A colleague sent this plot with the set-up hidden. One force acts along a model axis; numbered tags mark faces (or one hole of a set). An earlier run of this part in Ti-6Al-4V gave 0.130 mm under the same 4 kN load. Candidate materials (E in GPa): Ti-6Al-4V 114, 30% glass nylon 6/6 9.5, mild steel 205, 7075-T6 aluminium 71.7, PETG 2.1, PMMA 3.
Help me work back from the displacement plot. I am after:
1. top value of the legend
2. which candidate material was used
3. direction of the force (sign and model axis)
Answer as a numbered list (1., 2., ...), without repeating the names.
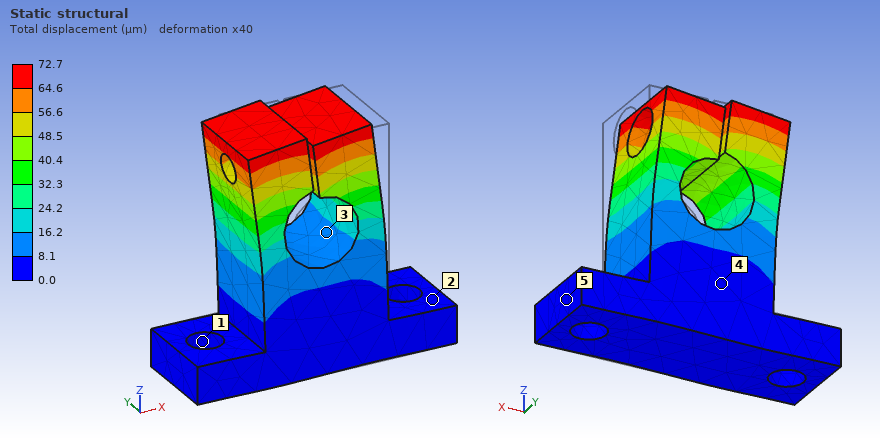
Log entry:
1. 72.7 µm
2. mild steel
3. -X
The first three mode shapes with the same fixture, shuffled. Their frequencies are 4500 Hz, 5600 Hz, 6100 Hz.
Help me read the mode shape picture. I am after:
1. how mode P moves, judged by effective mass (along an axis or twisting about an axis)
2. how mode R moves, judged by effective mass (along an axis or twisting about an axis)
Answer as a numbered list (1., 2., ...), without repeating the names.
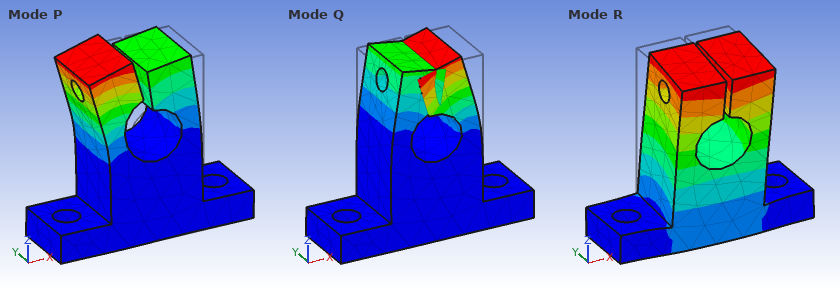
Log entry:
1. along X
2. along Y
